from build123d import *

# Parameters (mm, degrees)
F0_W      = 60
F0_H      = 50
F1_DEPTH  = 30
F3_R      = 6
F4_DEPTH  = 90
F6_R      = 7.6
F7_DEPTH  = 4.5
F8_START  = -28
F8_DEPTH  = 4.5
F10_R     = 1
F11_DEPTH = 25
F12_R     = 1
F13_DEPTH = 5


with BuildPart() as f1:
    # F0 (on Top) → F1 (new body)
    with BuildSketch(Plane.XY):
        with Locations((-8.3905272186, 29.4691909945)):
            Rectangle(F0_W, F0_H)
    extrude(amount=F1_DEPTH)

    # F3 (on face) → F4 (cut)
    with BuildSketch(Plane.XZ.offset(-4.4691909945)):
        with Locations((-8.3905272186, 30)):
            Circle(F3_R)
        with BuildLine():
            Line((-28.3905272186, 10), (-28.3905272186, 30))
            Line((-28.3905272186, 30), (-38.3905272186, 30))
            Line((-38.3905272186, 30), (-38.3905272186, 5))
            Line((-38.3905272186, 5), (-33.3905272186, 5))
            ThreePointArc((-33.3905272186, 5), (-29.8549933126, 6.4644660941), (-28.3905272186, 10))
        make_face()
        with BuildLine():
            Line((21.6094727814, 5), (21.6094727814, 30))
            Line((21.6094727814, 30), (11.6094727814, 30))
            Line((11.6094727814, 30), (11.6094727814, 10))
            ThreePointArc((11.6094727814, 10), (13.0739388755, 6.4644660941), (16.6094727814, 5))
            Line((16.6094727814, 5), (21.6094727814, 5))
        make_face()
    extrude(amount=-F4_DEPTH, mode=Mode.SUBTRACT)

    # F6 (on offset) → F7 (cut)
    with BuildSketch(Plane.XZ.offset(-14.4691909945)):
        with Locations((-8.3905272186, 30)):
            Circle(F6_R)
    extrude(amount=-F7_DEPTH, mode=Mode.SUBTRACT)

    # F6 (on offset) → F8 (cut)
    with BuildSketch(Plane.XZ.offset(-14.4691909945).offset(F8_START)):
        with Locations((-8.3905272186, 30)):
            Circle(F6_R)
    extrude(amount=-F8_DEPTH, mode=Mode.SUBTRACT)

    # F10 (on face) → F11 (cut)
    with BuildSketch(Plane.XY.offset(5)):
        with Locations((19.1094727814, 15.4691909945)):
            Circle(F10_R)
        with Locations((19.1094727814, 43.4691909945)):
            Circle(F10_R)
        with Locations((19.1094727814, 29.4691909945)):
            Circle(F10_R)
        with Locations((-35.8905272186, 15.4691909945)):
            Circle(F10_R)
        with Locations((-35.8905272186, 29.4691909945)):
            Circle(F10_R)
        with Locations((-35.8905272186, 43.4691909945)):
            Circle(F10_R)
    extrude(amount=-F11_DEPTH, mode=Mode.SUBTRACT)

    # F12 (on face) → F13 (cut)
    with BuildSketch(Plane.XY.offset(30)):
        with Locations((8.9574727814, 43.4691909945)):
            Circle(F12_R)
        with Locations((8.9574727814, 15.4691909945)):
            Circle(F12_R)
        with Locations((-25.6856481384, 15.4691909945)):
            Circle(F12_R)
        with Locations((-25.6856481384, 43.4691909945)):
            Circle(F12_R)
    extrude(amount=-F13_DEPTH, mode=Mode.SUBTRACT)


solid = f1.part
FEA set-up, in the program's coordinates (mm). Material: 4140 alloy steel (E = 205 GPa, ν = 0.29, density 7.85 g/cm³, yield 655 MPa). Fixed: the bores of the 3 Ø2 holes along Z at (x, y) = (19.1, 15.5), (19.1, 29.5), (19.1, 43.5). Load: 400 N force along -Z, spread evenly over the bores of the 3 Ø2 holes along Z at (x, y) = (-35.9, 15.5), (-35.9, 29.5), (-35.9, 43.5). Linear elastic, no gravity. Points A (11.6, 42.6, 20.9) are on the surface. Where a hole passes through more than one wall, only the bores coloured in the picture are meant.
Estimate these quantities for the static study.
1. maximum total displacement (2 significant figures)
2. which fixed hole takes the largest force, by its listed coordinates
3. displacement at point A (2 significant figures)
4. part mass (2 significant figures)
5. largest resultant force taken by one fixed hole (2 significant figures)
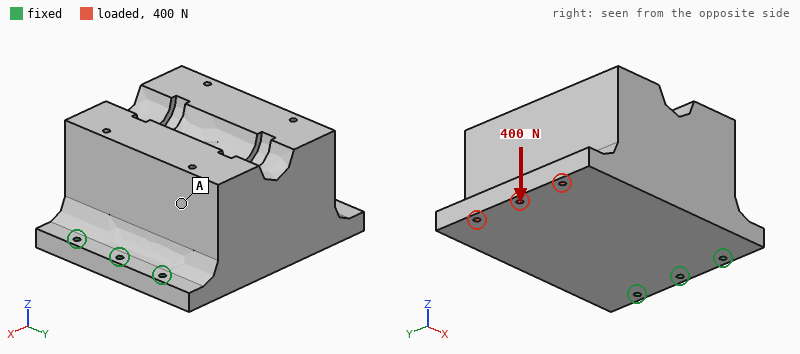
0.12 mm
(19.1, 29.5)
0.039 mm
490 g
200 N
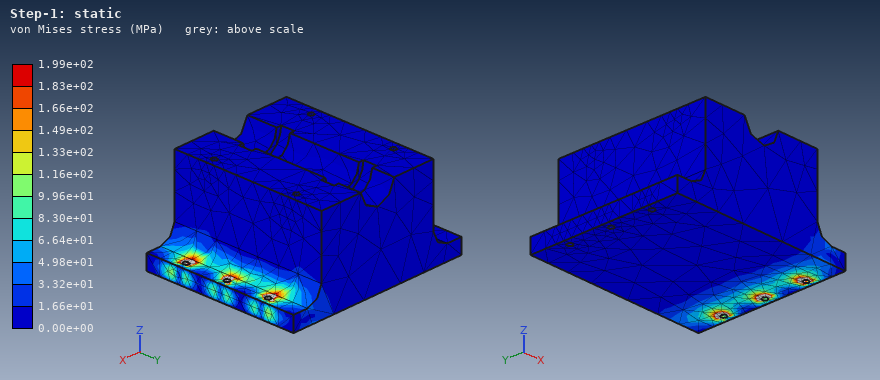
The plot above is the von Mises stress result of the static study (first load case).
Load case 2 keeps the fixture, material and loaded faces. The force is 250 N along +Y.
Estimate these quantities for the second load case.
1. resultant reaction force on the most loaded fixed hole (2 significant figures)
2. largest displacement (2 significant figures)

480 N
3.5 µm
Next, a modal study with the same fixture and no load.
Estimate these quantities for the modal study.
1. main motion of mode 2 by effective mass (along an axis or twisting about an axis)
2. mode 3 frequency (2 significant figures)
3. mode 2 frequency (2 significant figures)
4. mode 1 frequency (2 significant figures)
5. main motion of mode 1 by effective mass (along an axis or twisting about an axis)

along Y
4100 Hz
3300 Hz
730 Hz
along Z
